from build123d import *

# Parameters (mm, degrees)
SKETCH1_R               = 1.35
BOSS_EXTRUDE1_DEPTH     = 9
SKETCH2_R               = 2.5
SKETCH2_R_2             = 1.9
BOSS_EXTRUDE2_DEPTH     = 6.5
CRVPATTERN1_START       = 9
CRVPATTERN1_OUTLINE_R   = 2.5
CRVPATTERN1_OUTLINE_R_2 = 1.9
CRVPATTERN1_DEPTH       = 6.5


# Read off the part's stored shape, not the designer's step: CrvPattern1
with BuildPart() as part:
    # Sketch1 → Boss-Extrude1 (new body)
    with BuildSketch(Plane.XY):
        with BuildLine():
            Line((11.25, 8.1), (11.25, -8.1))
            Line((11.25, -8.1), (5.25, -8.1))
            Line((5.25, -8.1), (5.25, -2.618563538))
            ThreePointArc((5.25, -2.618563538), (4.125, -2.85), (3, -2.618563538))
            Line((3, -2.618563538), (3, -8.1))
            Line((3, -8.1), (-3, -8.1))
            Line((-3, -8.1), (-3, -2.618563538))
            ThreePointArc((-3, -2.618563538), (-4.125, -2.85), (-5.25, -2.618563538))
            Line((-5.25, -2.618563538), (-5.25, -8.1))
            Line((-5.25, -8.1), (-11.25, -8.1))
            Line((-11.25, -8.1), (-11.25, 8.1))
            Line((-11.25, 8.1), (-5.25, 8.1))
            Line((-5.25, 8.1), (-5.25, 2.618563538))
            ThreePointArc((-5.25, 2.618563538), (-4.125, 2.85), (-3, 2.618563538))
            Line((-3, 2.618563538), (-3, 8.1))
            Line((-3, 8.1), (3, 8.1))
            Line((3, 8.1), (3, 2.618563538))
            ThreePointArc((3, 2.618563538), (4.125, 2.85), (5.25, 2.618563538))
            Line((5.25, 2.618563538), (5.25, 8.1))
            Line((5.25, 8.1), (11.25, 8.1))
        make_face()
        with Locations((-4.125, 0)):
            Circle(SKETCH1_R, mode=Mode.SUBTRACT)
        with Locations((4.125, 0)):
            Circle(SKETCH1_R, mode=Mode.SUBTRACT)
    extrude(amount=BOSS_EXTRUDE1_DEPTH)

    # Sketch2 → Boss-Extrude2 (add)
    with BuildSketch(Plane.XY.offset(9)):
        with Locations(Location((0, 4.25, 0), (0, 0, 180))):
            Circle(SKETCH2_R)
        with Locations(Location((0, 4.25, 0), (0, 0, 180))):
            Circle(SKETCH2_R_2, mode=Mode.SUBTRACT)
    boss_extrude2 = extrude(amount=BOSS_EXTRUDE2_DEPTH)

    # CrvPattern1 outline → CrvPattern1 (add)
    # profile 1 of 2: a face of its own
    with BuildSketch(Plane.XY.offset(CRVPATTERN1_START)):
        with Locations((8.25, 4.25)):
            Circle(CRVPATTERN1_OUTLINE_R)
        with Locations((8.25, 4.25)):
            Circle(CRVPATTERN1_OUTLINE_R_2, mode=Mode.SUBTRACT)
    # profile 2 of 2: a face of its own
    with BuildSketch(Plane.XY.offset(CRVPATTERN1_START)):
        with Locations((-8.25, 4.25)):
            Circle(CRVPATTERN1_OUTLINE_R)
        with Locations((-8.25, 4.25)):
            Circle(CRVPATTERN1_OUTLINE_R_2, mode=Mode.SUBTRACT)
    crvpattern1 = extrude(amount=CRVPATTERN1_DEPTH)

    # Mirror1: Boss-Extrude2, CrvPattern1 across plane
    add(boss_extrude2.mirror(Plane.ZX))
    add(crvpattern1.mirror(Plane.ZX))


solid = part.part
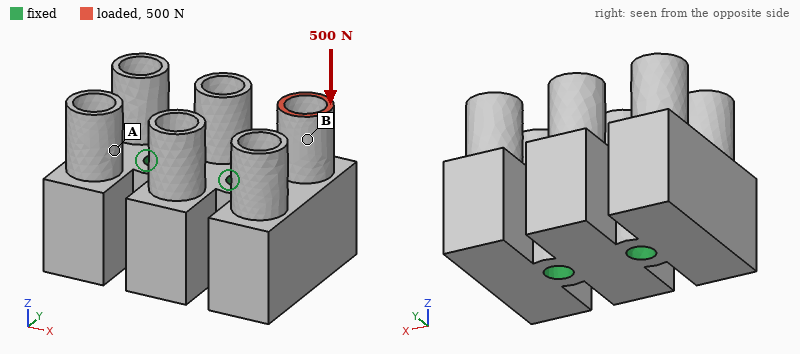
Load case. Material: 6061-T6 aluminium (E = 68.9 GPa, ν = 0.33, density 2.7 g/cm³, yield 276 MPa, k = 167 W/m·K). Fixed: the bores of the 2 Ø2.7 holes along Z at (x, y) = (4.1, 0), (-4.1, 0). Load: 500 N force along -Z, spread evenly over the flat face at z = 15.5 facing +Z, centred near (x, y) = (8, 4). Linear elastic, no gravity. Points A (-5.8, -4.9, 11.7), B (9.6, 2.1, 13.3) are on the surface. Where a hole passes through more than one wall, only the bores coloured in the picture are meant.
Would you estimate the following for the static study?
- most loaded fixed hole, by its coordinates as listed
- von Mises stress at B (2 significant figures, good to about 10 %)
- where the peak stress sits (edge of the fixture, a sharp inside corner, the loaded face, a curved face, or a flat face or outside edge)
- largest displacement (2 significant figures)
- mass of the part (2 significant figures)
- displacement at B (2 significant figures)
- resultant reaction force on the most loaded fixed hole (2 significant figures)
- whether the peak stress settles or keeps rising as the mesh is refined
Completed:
(4.1, 0)
60 MPa
edge of the fixture
13 µm
8.3 g
8.2 µm
500 N
keeps rising
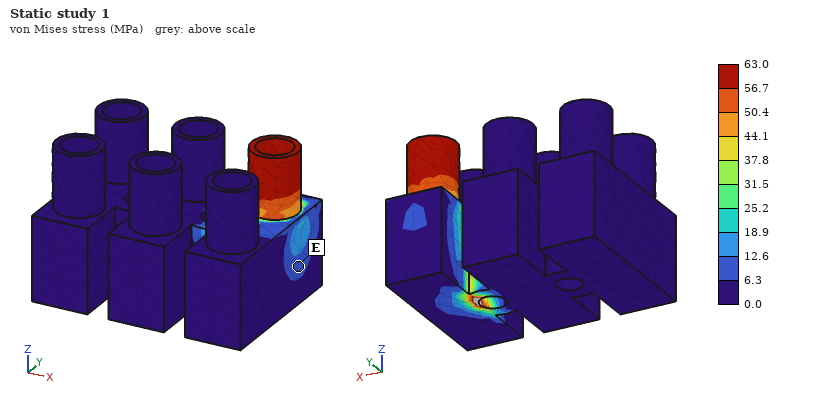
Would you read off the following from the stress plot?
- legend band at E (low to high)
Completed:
6.3 to 12.6 MPa
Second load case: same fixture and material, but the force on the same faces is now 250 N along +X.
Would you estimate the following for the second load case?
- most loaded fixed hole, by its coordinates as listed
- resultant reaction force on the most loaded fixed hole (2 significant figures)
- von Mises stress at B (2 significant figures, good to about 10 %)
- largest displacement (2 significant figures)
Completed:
(4.1, 0)
240 N
92 MPa
56 µm
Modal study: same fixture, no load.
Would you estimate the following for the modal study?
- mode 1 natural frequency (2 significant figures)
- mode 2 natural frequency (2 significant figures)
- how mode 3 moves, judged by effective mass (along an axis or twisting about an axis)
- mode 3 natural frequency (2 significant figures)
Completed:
25 kHz
26 kHz
twisting about X
38 kHz
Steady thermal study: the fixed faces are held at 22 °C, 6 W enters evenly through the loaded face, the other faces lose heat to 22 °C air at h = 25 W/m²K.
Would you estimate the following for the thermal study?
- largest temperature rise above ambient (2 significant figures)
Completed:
34 K
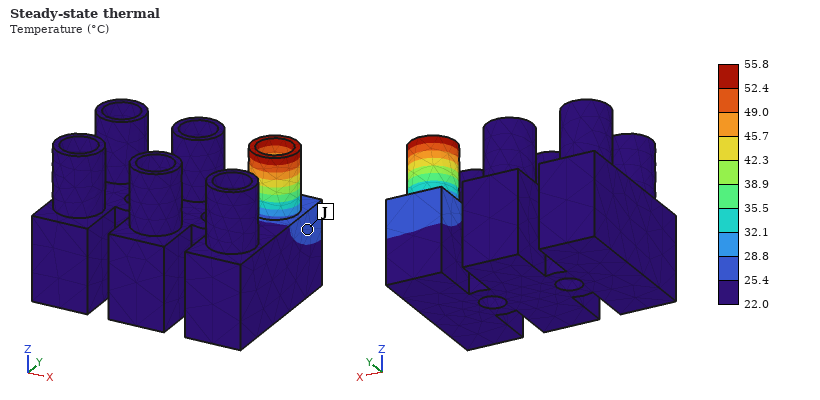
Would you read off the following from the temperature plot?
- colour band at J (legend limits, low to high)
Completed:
25.4 to 28.8 °C
